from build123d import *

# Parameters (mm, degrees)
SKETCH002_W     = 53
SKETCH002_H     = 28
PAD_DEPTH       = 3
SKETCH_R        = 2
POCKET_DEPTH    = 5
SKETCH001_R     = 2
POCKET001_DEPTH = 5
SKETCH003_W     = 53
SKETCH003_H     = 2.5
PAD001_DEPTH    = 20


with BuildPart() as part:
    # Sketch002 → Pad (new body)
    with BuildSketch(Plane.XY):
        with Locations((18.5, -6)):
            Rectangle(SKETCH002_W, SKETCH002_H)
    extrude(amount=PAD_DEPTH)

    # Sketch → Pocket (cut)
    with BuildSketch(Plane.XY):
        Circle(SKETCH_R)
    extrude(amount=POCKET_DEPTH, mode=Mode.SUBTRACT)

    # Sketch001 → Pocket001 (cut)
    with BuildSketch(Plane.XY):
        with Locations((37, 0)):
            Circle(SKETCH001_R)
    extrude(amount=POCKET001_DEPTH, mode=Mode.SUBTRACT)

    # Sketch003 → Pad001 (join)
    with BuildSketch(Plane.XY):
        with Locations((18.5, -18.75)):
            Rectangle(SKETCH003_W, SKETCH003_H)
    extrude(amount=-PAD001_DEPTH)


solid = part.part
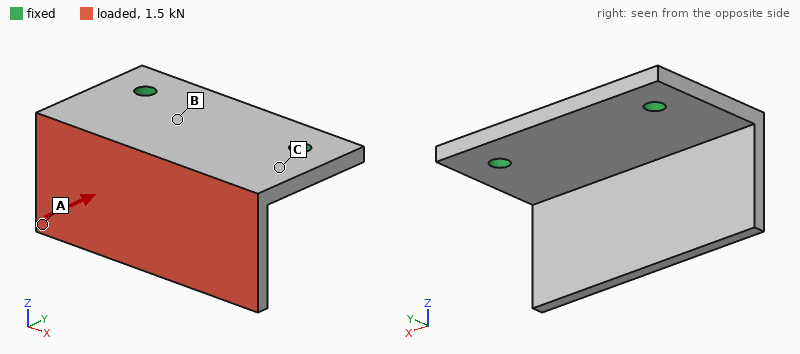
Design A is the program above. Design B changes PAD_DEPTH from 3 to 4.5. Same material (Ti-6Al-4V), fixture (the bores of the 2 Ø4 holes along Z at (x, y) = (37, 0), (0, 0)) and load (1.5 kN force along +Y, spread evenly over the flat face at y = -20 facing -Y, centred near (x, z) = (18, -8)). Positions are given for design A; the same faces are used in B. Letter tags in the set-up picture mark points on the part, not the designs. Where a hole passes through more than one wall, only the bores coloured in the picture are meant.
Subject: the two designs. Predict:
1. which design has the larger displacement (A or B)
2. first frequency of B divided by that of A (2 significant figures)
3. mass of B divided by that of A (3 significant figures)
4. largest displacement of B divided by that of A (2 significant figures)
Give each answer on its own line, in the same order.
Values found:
A
1.5
1.31
0.50
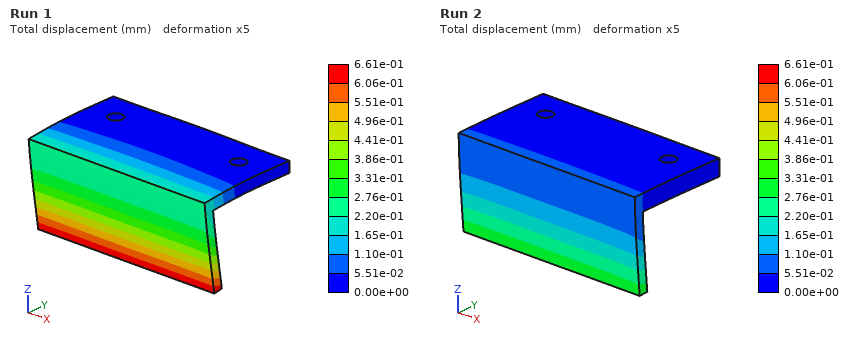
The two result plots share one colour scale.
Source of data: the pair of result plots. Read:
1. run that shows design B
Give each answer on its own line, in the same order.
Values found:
Run 2
